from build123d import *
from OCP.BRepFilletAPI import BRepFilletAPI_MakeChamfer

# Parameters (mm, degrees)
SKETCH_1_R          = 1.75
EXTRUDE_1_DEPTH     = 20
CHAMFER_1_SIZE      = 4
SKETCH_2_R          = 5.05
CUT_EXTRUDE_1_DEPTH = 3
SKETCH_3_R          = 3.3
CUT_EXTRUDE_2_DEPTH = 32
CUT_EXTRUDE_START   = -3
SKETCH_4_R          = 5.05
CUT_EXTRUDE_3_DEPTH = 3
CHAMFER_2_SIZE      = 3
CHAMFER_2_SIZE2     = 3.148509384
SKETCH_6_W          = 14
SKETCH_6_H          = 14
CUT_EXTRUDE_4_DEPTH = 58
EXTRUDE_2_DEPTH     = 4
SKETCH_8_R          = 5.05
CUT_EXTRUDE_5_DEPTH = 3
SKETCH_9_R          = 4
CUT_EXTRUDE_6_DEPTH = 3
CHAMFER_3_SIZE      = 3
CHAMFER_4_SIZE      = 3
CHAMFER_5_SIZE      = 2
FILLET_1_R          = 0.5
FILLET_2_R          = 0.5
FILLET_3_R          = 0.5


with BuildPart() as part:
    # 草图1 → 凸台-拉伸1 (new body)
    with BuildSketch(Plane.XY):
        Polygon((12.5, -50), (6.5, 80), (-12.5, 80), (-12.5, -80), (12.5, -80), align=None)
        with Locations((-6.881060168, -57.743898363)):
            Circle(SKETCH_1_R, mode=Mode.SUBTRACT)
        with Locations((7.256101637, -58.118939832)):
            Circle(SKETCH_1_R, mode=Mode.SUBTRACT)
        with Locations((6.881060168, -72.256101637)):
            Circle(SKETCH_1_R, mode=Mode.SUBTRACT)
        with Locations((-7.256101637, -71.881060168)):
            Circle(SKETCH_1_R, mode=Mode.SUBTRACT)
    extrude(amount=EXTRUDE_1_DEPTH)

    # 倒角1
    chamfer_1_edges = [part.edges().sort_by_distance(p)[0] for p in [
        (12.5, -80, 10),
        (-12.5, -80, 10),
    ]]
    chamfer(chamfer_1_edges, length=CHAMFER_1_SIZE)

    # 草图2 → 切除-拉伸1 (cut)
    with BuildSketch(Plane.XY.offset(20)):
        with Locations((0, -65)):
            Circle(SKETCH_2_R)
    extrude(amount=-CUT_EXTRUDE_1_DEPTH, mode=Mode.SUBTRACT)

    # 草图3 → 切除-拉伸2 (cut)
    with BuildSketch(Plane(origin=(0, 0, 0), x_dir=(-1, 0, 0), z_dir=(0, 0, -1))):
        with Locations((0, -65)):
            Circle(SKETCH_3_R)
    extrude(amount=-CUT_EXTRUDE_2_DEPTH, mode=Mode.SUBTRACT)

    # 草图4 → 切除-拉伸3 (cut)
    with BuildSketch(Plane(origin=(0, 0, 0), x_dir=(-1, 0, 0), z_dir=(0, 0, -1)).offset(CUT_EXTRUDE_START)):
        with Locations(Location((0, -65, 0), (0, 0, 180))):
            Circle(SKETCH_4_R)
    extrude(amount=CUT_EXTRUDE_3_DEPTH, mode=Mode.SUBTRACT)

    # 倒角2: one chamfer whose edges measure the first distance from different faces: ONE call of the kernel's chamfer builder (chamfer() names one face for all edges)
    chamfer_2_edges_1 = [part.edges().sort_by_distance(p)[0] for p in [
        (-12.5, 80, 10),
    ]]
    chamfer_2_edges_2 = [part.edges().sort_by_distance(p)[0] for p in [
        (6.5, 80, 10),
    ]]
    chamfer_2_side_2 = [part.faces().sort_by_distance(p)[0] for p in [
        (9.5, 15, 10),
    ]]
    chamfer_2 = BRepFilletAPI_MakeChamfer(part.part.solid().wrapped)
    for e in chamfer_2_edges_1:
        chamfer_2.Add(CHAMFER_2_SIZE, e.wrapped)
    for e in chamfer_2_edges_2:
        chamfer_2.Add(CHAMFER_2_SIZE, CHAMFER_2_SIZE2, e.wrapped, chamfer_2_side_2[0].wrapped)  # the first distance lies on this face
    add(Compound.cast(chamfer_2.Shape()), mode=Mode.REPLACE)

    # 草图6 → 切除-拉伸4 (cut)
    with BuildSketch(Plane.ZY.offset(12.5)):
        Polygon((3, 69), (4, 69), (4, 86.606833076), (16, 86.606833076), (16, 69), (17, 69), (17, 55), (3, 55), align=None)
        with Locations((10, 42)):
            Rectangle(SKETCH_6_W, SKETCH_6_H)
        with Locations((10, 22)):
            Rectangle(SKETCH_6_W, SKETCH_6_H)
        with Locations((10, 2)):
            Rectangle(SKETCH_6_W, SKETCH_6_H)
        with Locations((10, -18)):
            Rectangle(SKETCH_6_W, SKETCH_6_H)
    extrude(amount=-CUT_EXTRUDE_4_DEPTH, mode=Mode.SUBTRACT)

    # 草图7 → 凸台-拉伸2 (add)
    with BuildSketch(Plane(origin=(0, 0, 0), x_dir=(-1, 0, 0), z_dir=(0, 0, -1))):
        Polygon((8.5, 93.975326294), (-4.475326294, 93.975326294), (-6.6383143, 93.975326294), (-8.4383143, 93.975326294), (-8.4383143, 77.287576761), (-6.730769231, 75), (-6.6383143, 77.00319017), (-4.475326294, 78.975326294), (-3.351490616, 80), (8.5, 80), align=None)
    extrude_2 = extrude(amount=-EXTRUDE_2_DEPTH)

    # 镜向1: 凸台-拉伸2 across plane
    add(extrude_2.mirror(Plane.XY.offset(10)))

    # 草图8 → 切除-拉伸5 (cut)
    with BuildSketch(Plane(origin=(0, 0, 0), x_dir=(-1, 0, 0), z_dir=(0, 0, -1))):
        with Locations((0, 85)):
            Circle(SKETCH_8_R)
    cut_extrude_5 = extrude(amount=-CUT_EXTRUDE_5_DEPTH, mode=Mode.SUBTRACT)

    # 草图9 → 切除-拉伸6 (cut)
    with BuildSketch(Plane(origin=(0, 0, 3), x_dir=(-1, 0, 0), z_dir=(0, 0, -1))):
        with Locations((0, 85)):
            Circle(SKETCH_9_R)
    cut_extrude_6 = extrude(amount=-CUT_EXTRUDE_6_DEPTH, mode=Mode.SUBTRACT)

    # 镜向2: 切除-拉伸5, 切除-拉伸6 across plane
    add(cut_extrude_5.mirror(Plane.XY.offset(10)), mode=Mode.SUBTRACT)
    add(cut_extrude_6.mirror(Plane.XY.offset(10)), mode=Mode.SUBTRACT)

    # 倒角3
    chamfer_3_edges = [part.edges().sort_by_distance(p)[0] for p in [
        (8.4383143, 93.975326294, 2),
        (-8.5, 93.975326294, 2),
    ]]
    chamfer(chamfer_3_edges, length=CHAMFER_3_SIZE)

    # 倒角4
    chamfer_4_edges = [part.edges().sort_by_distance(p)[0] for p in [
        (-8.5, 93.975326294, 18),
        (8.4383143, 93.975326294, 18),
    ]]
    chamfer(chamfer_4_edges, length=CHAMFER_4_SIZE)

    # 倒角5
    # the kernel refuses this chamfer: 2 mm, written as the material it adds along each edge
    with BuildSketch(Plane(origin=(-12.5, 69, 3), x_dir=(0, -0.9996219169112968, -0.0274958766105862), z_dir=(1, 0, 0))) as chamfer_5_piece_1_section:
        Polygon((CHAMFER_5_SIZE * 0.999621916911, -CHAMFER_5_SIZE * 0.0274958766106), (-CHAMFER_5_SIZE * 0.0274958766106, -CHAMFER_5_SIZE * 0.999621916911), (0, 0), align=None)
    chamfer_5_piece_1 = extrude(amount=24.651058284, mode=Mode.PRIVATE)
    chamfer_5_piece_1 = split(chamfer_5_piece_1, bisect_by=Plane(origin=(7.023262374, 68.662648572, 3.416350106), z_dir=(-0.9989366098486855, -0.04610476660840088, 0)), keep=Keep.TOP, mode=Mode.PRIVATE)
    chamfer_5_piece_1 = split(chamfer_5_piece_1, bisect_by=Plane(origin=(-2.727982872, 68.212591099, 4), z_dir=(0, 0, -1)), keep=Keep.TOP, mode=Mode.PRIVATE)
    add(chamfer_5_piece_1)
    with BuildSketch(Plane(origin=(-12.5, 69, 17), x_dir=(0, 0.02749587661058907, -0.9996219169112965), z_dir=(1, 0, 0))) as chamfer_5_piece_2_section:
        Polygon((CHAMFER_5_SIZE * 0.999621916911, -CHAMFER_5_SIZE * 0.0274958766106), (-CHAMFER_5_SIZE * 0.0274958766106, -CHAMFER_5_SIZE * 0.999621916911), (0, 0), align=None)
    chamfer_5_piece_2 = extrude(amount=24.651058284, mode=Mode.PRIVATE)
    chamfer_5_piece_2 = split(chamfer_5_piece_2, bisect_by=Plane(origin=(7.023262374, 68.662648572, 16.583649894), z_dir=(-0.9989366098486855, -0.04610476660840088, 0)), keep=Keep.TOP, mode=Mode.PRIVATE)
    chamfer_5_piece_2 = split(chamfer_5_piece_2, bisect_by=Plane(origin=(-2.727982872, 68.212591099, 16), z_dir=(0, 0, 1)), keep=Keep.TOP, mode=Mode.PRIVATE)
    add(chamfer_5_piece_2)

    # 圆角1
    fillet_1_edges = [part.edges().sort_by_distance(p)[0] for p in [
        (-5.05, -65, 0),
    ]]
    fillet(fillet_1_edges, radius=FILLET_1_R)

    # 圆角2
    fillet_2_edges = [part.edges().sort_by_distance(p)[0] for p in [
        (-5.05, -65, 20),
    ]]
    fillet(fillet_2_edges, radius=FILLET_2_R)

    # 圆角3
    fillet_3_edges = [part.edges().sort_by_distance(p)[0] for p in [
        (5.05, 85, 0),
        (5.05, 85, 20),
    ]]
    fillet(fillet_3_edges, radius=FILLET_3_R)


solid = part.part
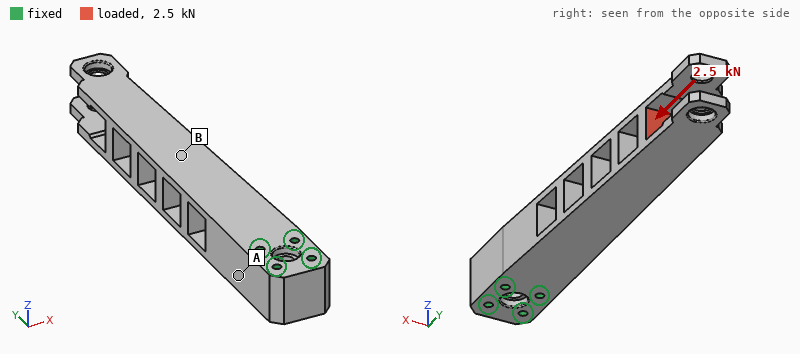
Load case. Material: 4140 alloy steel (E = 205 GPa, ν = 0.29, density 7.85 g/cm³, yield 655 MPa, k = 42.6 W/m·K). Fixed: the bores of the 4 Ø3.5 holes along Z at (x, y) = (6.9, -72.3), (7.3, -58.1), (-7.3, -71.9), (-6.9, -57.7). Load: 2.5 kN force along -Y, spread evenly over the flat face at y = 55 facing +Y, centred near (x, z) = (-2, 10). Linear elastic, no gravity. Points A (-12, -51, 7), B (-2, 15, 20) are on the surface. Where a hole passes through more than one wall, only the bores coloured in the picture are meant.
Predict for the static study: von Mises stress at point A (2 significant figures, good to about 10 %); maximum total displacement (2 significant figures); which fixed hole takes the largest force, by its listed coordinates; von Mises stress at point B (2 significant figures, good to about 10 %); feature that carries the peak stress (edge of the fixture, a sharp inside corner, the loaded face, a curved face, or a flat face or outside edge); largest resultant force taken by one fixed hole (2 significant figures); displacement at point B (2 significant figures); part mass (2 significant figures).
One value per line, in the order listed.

6.5 MPa
27 µm
(-6.9, -57.7)
19 MPa
a flat face or outside edge
1.5 kN
6.6 µm
370 g
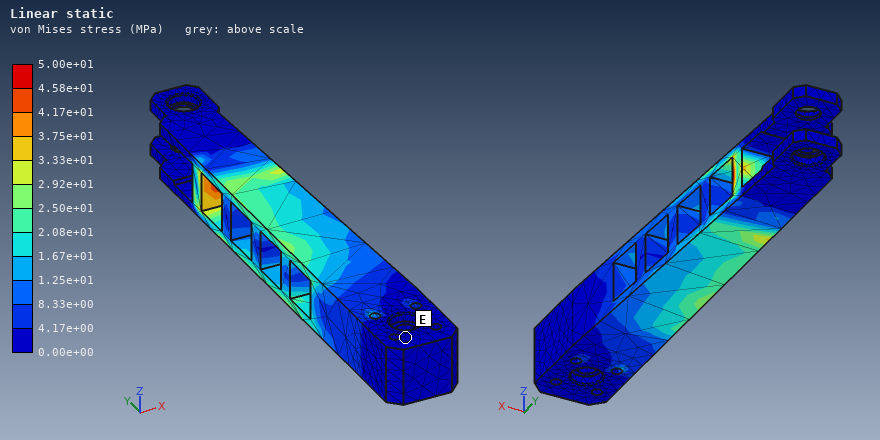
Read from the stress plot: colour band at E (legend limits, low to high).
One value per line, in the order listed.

0.00e+00 to 4.17e+00 MPa
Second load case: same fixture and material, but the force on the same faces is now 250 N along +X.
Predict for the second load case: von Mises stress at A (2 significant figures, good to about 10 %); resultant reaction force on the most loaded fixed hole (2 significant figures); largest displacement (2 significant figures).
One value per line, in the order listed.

11 MPa
1.6 kN
86 µm
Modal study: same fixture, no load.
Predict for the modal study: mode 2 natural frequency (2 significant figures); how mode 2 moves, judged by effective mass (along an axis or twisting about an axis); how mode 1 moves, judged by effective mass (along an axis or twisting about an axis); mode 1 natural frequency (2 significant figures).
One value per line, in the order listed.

1100 Hz
along X
along Z
950 Hz
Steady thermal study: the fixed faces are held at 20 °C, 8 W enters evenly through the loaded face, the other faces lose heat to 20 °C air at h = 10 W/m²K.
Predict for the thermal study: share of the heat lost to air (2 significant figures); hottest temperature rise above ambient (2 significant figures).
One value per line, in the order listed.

61 %
62 K
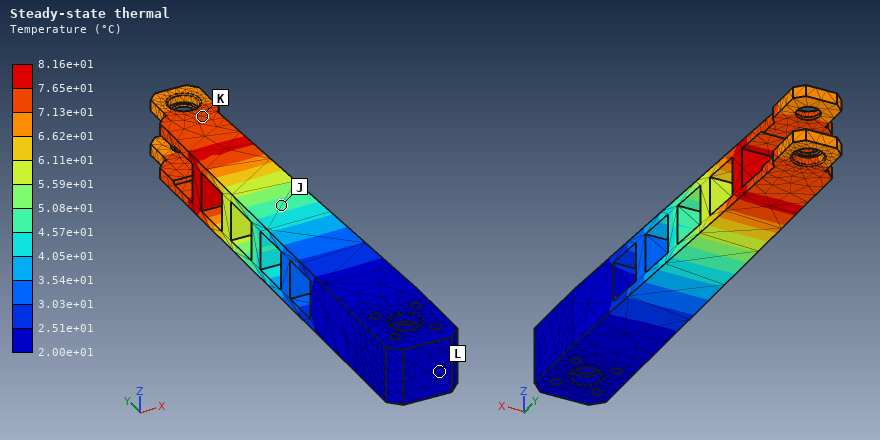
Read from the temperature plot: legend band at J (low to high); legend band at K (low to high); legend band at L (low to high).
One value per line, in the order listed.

4.57e+01 to 5.08e+01 °C
7.13e+01 to 7.65e+01 °C
2.00e+01 to 2.51e+01 °C
